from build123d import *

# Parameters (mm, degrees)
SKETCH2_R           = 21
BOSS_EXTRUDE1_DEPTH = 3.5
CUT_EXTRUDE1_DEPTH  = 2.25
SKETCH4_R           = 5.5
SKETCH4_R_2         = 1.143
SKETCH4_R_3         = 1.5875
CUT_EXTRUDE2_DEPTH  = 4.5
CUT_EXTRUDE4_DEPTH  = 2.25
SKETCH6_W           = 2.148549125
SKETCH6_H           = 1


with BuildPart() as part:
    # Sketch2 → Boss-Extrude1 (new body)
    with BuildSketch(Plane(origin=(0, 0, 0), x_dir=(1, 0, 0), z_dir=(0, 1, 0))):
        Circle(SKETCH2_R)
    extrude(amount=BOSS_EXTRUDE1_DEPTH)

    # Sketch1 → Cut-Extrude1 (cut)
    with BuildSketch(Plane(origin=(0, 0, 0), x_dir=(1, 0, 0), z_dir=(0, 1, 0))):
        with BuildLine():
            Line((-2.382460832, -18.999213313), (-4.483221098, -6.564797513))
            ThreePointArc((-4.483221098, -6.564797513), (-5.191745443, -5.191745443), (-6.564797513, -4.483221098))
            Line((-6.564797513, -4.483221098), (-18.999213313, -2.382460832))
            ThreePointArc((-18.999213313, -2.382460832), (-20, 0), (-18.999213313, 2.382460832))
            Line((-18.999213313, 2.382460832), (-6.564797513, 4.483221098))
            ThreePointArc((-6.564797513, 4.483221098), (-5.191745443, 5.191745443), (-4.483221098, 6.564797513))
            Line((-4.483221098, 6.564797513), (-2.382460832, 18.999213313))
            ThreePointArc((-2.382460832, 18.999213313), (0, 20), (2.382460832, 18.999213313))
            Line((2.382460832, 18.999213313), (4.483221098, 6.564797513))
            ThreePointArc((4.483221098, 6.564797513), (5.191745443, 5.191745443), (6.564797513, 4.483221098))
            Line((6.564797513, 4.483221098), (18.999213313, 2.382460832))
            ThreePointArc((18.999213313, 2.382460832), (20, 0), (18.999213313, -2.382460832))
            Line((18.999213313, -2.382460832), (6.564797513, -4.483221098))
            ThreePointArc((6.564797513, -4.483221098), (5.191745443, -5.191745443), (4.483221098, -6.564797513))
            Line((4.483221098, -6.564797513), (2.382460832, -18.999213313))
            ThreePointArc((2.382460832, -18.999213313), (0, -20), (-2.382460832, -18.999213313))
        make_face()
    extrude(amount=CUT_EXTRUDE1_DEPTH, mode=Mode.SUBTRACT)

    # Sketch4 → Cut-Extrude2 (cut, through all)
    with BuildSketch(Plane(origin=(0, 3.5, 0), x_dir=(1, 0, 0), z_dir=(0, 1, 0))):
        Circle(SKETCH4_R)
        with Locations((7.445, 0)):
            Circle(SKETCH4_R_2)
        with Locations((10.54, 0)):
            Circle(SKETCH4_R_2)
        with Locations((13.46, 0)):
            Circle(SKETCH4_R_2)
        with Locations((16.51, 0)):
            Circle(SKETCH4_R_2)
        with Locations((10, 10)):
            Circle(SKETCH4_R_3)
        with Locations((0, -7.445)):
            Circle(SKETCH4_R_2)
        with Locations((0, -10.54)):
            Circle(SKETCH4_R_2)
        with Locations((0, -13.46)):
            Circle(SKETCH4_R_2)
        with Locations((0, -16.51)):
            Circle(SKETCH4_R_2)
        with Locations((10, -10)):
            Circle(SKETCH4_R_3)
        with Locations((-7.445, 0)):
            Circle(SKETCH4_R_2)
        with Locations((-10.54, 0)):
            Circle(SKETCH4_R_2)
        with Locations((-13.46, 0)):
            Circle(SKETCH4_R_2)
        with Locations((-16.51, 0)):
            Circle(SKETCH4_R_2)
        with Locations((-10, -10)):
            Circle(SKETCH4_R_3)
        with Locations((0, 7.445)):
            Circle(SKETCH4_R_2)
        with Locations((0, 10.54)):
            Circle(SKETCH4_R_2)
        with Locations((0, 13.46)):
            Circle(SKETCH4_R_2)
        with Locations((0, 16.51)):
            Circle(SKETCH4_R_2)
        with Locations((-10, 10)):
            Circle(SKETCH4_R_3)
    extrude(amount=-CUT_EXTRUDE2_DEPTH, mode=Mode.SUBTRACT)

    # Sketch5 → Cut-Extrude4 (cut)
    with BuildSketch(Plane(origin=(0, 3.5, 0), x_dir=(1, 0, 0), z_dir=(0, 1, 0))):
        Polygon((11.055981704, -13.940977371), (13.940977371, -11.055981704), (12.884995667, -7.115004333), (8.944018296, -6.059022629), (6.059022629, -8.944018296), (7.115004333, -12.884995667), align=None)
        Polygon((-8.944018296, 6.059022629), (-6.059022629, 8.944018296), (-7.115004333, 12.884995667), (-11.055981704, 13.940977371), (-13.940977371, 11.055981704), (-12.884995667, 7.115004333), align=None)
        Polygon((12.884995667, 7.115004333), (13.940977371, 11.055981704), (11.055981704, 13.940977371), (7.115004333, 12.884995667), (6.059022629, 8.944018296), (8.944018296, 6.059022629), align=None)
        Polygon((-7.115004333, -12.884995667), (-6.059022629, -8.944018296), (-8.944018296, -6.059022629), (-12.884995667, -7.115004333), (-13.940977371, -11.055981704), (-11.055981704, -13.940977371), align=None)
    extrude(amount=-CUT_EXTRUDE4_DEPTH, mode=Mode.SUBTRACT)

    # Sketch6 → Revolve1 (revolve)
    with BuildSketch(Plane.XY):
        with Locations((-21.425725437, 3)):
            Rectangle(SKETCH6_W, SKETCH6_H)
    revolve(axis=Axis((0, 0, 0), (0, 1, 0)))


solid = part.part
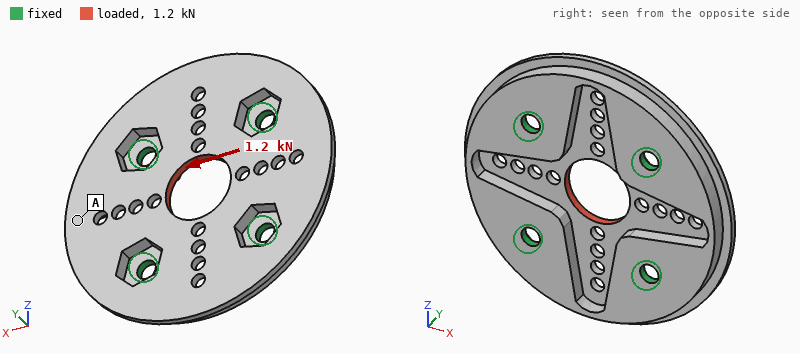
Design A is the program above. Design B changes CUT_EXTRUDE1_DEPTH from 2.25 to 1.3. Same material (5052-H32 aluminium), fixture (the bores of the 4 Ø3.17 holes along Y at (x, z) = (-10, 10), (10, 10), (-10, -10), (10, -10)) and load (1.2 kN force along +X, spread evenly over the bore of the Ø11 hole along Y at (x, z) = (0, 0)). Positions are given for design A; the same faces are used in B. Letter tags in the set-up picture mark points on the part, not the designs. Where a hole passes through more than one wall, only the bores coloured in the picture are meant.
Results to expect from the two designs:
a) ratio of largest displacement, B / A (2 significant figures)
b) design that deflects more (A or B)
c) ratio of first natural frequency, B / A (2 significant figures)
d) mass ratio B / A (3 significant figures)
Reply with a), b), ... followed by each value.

a) 0.59
b) A
c) 0.99
d) 1.10
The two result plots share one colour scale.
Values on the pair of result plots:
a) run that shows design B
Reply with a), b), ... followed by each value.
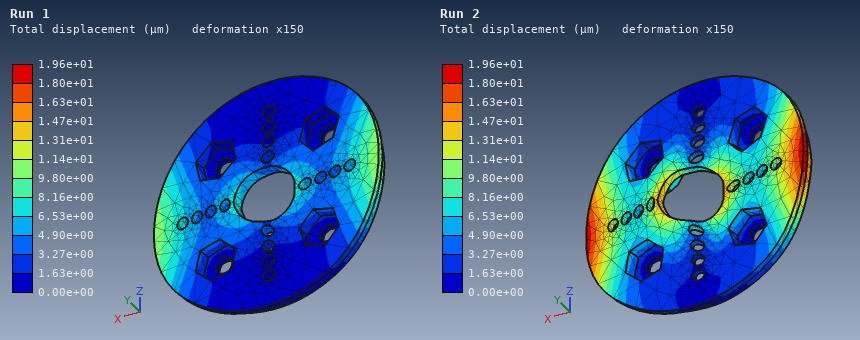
a) Run 1
